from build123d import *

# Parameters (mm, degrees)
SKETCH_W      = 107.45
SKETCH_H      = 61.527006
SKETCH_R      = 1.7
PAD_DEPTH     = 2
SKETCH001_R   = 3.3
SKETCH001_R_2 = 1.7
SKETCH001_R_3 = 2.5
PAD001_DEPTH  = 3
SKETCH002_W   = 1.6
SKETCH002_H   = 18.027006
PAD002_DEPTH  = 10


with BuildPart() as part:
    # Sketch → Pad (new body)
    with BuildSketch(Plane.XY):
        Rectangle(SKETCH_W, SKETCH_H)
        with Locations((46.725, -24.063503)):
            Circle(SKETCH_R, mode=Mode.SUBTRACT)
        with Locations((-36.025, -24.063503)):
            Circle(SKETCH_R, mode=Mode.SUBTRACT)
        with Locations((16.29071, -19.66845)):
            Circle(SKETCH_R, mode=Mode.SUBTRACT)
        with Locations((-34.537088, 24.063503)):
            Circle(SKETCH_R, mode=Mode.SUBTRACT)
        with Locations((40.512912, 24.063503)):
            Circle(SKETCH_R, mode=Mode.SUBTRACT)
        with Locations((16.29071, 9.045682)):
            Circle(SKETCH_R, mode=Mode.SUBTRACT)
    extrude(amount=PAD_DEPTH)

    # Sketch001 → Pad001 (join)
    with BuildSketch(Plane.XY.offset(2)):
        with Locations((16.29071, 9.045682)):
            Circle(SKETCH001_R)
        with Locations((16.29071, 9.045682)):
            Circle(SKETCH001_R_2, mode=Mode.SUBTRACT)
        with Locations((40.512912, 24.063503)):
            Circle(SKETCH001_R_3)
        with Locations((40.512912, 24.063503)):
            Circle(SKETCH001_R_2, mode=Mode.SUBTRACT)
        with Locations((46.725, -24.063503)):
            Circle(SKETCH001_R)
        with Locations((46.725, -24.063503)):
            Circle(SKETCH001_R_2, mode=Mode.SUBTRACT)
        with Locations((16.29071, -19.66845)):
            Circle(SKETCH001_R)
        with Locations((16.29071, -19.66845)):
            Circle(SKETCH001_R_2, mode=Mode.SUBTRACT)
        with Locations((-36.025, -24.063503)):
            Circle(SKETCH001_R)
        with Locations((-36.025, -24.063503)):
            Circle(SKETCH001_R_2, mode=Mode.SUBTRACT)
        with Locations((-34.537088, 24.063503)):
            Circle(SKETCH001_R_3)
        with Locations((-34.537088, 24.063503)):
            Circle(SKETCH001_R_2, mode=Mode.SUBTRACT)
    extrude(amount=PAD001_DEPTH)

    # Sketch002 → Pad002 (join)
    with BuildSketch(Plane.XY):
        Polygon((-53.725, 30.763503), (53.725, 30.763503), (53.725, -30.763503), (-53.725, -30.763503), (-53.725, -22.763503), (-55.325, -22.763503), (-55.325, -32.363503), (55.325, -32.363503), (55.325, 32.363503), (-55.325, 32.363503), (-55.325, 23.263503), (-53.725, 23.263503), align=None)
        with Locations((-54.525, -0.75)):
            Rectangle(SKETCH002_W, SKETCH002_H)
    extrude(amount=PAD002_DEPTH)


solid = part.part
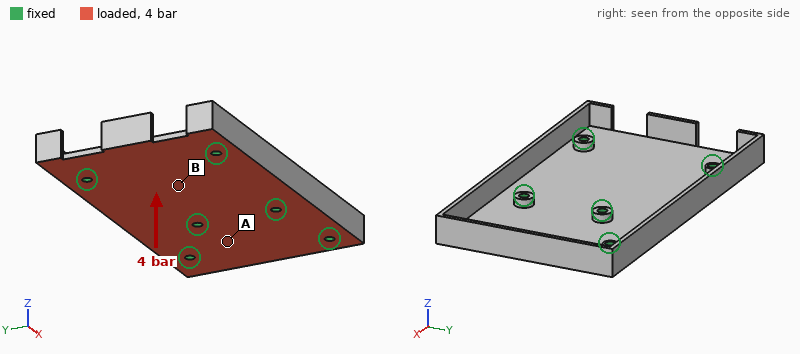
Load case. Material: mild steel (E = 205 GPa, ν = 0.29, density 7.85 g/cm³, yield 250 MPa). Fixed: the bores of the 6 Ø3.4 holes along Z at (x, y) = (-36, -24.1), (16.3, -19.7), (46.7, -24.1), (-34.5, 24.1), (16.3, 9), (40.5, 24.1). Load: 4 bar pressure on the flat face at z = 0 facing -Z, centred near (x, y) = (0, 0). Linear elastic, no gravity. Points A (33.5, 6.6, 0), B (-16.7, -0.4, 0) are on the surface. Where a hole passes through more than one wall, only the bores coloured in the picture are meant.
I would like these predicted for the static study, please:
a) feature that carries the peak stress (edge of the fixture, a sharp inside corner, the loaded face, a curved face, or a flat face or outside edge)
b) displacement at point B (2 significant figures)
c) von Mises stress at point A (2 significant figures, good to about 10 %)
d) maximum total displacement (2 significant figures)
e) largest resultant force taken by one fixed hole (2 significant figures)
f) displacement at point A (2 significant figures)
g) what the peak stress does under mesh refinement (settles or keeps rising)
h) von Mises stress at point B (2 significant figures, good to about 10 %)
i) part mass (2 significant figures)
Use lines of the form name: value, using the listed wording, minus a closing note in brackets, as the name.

feature that carries the peak stress: edge of the fixture
displacement at point B: 65 µm
von Mises stress at point A: 19 MPa
maximum total displacement: 65 µm
largest resultant force taken by one fixed hole: 630 N
displacement at point A: 12 µm
what the peak stress does under mesh refinement: keeps rising
von Mises stress at point B: 54 MPa
part mass: 150 g
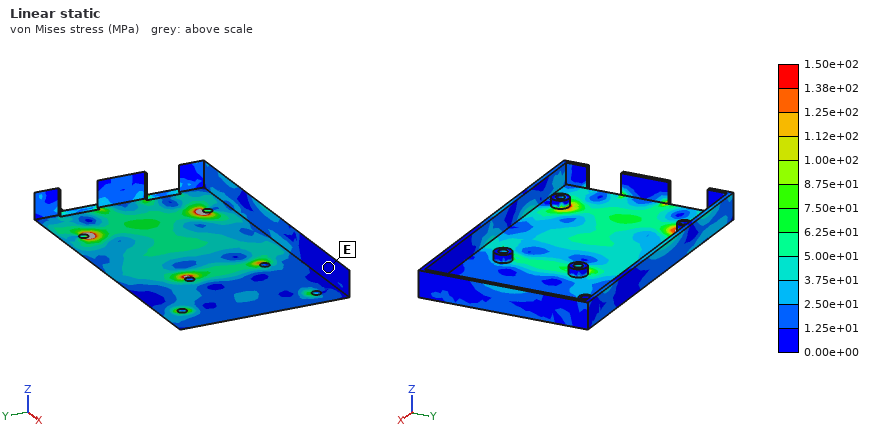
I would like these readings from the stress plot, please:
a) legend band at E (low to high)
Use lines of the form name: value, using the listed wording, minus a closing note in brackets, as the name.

legend band at E: 0.00e+00 to 1.25e+01 MPa
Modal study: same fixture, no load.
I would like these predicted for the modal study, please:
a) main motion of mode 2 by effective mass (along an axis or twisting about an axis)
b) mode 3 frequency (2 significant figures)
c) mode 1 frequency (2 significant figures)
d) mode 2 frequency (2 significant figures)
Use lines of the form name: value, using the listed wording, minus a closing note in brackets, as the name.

main motion of mode 2 by effective mass: along Z
mode 3 frequency: 4800 Hz
mode 1 frequency: 3100 Hz
mode 2 frequency: 3800 Hz
